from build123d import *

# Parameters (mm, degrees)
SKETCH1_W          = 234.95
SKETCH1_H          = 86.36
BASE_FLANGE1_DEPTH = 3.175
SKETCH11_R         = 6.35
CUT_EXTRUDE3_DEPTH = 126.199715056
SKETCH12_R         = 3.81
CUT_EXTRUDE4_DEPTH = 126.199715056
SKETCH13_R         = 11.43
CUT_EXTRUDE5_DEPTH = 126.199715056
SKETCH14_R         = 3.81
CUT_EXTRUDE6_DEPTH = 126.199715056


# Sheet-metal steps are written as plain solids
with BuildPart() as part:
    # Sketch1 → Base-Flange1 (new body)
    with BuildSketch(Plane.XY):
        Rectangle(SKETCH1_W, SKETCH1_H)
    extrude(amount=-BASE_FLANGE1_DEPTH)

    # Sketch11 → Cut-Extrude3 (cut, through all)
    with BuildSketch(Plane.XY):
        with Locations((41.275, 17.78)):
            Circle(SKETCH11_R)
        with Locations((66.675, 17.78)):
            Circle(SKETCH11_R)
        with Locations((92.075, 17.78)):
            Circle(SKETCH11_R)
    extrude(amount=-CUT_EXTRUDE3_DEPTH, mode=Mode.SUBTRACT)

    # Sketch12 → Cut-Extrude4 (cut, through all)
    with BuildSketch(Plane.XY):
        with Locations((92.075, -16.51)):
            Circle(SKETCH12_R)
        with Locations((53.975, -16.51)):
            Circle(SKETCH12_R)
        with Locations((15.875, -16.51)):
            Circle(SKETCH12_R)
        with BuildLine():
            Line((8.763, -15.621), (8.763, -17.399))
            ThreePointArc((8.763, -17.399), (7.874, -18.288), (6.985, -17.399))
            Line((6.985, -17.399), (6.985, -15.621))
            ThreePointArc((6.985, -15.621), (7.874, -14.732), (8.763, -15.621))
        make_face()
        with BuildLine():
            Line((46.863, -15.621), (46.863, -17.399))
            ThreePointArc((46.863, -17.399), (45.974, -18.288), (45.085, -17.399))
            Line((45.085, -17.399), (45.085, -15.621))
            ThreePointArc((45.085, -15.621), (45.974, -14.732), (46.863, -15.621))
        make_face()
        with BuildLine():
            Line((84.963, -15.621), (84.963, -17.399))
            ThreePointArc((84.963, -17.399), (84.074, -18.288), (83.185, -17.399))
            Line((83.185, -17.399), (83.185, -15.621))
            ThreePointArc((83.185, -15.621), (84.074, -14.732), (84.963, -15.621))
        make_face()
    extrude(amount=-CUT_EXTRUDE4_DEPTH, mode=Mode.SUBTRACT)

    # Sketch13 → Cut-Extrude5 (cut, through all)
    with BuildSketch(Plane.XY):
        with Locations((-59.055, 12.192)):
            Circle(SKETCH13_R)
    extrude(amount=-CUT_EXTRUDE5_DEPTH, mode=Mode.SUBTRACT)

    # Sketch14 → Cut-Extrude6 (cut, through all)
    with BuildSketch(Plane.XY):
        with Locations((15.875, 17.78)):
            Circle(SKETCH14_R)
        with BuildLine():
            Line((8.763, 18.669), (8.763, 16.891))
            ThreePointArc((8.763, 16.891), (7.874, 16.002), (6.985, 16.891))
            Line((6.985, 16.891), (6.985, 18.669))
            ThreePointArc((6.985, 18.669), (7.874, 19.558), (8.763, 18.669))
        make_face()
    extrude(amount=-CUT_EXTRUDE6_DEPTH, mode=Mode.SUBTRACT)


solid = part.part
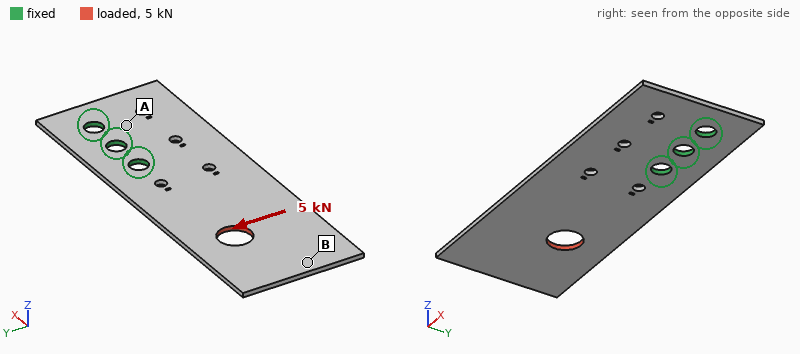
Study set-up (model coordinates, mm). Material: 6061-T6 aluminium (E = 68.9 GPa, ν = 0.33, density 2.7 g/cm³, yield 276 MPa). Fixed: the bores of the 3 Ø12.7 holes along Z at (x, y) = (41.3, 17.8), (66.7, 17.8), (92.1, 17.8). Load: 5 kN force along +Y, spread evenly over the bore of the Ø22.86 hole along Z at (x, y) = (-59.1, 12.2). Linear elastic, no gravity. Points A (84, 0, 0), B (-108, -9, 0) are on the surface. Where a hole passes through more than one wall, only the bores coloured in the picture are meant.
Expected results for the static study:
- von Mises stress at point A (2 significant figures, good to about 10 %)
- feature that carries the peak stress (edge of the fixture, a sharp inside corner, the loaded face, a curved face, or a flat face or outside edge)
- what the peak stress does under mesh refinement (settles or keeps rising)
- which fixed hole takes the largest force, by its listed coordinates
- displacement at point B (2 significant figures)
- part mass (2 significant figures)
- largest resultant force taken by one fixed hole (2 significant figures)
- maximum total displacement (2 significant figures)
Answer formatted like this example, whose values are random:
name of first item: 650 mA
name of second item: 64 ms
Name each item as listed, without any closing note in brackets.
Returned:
von Mises stress at point A: 78 MPa
feature that carries the peak stress: edge of the fixture
what the peak stress does under mesh refinement: keeps rising
which fixed hole takes the largest force, by its listed coordinates: (41.3, 17.8)
displacement at point B: 0.70 mm
part mass: 170 g
largest resultant force taken by one fixed hole: 13 kN
maximum total displacement: 0.77 mm
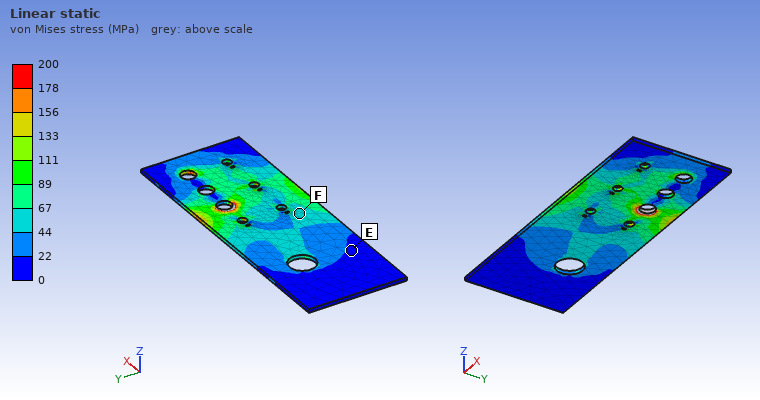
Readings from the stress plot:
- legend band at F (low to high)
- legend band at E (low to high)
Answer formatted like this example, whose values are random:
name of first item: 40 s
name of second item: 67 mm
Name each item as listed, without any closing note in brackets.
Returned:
legend band at F: 44 to 67 MPa
legend band at E: 0 to 22 MPa
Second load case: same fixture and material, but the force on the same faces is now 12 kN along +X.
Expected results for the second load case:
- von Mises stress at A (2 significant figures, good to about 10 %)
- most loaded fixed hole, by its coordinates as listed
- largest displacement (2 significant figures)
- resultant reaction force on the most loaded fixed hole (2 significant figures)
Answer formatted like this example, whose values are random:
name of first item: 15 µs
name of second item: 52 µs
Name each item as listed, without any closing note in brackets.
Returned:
von Mises stress at A: 22 MPa
most loaded fixed hole, by its coordinates as listed: (41.3, 17.8)
largest displacement: 0.15 mm
resultant reaction force on the most loaded fixed hole: 8.5 kN
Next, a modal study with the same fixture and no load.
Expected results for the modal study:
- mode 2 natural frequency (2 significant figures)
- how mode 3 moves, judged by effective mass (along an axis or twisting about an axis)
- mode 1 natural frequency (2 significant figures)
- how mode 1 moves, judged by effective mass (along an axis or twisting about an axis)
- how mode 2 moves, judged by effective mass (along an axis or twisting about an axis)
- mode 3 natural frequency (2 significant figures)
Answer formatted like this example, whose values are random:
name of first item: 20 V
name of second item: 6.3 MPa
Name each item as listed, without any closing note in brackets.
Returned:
mode 2 natural frequency: 350 Hz
how mode 3 moves, judged by effective mass: along Z
mode 1 natural frequency: 100 Hz
how mode 1 moves, judged by effective mass: along Z
how mode 2 moves, judged by effective mass: twisting about X
mode 3 natural frequency: 600 Hz
